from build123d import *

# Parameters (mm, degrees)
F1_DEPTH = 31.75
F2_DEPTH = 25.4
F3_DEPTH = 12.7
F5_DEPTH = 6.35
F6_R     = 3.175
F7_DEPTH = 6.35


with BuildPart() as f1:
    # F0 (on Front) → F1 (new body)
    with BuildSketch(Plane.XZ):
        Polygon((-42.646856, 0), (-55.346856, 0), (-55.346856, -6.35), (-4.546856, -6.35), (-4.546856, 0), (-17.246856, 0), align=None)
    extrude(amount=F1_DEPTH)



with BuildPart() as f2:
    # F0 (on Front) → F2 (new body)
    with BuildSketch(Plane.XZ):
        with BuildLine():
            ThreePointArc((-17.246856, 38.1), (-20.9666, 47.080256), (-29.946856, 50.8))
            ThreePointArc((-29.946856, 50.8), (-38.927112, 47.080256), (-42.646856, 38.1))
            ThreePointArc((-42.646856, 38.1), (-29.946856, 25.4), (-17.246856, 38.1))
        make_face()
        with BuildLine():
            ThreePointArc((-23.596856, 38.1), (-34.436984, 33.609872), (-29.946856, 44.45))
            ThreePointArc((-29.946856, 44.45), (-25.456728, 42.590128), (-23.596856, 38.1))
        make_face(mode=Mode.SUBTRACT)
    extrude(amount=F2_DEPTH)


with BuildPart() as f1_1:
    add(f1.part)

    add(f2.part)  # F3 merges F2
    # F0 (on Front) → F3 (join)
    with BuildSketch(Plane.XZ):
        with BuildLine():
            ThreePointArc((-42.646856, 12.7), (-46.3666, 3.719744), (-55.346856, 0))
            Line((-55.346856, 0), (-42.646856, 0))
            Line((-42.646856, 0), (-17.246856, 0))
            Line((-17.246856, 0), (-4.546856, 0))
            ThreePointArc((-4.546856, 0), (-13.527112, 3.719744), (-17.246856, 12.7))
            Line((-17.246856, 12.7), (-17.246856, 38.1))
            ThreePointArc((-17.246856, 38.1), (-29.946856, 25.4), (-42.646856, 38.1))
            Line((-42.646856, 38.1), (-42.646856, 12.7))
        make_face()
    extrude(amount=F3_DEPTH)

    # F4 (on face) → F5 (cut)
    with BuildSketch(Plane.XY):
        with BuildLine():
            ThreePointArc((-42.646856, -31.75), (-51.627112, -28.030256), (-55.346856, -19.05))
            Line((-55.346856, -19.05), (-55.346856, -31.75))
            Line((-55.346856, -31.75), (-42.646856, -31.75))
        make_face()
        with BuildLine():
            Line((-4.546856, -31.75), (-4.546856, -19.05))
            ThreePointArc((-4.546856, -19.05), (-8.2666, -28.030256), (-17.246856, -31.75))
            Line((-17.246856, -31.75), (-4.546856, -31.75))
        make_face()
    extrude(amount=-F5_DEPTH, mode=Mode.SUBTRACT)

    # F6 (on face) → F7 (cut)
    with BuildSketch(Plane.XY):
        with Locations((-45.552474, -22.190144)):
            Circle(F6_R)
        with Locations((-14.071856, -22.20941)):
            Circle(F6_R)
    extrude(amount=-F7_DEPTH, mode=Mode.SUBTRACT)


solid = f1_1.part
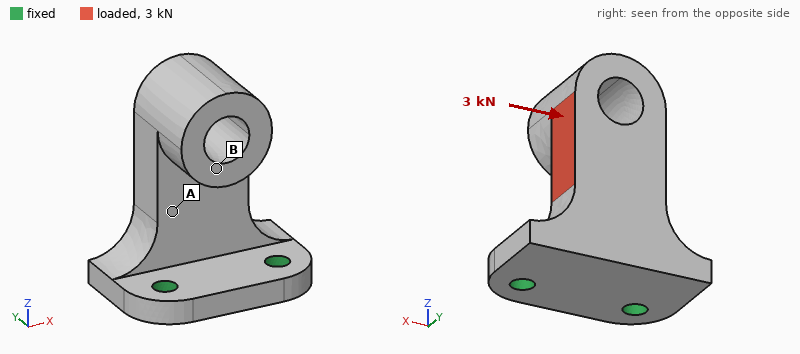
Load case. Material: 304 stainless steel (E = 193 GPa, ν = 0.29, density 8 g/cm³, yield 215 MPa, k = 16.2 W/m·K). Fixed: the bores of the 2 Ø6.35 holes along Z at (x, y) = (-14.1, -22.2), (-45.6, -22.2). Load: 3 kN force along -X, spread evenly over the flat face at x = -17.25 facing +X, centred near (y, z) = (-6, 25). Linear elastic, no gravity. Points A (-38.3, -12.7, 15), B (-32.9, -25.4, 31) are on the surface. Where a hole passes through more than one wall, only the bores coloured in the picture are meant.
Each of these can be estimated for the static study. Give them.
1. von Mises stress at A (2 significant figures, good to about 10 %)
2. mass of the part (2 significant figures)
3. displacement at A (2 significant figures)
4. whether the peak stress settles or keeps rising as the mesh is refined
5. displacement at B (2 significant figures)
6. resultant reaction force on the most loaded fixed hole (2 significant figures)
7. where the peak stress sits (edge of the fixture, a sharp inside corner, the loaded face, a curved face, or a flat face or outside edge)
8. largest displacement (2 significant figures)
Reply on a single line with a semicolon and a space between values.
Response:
30 MPa; 230 g; 19 µm; keeps rising; 37 µm; 3.2 kN; edge of the fixture; 56 µm
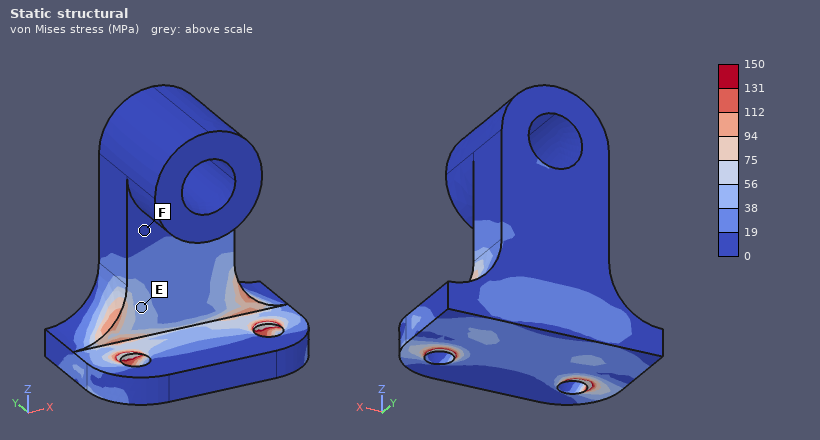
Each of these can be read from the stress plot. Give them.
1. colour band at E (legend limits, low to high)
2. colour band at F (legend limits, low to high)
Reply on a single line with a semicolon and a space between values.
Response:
38 to 56 MPa; 0 to 19 MPa
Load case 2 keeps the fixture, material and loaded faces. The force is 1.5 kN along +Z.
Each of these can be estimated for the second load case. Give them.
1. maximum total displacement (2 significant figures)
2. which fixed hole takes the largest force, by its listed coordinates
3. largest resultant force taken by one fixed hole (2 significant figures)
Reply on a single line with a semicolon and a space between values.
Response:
50 µm; (-14.1, -22.2); 1.3 kN
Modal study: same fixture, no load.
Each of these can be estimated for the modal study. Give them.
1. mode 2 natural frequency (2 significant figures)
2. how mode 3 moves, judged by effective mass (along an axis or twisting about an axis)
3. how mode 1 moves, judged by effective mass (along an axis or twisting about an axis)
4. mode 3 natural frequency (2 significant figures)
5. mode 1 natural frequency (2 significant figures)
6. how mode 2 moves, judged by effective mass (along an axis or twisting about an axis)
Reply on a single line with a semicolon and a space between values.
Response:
3300 Hz; along Z; along Y; 6300 Hz; 1400 Hz; along X
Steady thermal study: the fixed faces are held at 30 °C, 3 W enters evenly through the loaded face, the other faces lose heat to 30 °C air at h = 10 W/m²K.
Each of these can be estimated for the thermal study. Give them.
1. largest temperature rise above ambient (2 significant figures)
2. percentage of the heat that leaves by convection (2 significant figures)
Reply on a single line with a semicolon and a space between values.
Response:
21 K; 29 %
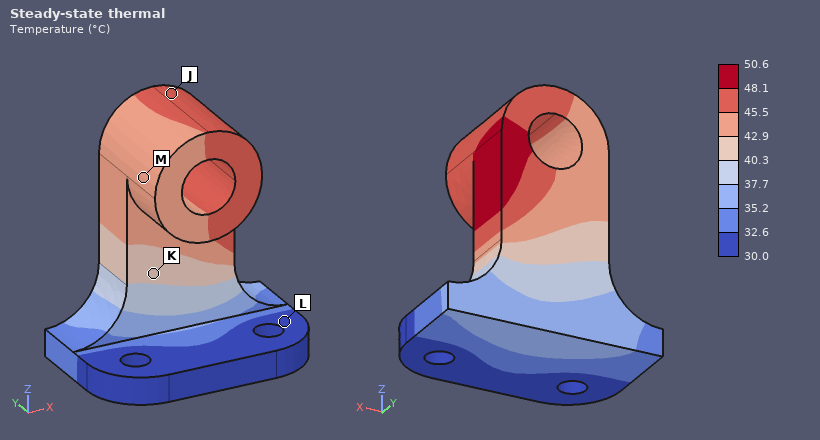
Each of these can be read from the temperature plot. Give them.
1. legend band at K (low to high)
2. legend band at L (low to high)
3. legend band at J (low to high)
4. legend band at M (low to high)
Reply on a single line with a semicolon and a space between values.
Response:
40.3 to 42.9 °C; 30.0 to 32.6 °C; 45.5 to 48.1 °C; 42.9 to 45.5 °C
